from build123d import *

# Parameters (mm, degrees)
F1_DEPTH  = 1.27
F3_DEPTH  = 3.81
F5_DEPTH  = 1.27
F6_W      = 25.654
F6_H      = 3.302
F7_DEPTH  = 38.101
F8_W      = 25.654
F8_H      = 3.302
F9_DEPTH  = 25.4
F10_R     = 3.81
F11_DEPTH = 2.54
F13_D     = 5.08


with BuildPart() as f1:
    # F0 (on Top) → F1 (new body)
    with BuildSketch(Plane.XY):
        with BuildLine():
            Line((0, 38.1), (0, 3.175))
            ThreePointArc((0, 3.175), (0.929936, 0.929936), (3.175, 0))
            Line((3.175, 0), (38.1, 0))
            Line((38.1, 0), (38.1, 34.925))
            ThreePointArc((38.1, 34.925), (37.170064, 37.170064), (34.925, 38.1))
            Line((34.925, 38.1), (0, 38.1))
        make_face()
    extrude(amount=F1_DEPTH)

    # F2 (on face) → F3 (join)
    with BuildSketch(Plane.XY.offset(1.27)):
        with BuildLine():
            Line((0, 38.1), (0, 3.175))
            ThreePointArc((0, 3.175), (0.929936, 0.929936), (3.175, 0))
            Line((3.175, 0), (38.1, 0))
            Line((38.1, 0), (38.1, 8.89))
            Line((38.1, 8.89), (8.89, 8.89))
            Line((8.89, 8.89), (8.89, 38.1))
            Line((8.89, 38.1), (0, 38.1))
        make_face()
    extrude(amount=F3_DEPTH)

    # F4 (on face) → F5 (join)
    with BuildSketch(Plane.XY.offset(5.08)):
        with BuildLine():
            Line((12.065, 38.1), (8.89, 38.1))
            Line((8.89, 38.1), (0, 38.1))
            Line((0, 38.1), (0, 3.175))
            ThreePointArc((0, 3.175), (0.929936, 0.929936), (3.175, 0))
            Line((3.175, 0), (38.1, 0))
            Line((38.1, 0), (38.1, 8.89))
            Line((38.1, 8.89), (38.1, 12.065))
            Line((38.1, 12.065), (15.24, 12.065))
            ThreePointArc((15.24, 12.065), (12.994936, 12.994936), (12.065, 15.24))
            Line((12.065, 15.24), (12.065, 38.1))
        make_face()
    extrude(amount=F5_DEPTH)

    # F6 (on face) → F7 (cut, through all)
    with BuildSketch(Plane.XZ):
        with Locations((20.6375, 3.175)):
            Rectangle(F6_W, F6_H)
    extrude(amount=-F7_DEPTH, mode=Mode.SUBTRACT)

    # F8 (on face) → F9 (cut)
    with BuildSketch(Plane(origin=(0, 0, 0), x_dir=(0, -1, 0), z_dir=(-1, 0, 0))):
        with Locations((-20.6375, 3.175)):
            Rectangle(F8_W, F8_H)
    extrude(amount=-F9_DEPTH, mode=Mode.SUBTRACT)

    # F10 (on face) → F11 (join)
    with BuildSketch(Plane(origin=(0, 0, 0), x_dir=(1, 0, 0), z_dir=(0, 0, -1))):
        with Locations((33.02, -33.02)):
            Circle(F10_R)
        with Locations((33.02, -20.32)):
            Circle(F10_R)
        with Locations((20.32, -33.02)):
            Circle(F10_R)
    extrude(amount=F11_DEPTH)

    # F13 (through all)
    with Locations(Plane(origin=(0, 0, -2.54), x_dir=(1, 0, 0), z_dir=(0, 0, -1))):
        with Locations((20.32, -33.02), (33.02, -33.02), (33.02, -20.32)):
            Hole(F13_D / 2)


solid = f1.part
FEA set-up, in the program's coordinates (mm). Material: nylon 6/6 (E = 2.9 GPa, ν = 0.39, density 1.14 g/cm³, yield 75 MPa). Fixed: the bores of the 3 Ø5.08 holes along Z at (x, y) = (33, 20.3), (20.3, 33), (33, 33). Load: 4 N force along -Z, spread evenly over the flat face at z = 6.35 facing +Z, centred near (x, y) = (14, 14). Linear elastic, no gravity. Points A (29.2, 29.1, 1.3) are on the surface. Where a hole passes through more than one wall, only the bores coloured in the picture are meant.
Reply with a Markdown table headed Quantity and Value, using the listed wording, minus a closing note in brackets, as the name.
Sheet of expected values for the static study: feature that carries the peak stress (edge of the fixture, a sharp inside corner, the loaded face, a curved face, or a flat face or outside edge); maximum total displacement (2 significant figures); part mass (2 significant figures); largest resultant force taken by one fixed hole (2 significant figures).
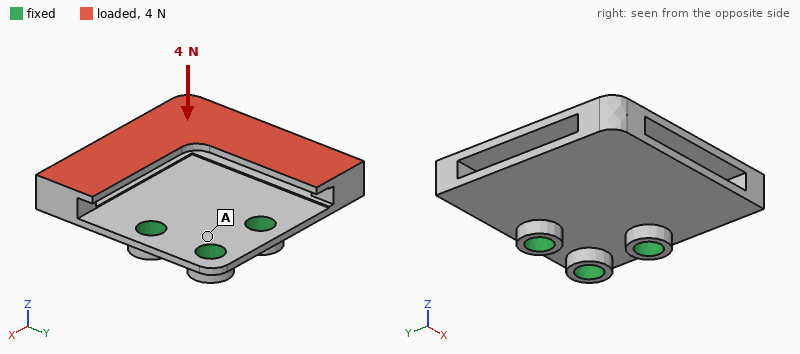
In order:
| Quantity | Value |
|---|---|
| feature that carries the peak stress | a flat face or outside edge |
| maximum total displacement | 0.58 mm |
| part mass | 4.2 g |
| largest resultant force taken by one fixed hole | 2.3 N |
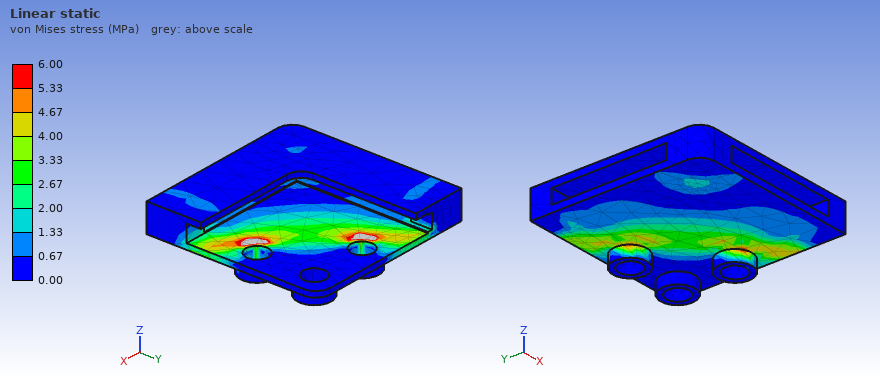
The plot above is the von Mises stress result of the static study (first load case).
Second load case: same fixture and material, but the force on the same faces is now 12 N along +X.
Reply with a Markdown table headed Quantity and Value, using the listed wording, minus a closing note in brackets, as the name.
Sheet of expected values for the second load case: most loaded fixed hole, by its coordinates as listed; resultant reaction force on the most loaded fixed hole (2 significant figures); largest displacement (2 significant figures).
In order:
| Quantity | Value |
|---|---|
| most loaded fixed hole, by its coordinates as listed | (33, 20.3) |
| resultant reaction force on the most loaded fixed hole | 11 N |
| largest displacement | 0.55 mm |
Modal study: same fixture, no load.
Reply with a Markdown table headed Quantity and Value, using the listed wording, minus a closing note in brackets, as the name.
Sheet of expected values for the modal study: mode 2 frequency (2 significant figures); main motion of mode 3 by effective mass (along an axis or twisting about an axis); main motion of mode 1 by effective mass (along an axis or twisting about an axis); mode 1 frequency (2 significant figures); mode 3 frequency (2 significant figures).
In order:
| Quantity | Value |
|---|---|
| mode 2 frequency | 750 Hz |
| main motion of mode 3 by effective mass | along Z |
| main motion of mode 1 by effective mass | along Z |
| mode 1 frequency | 300 Hz |
| mode 3 frequency | 1500 Hz |
